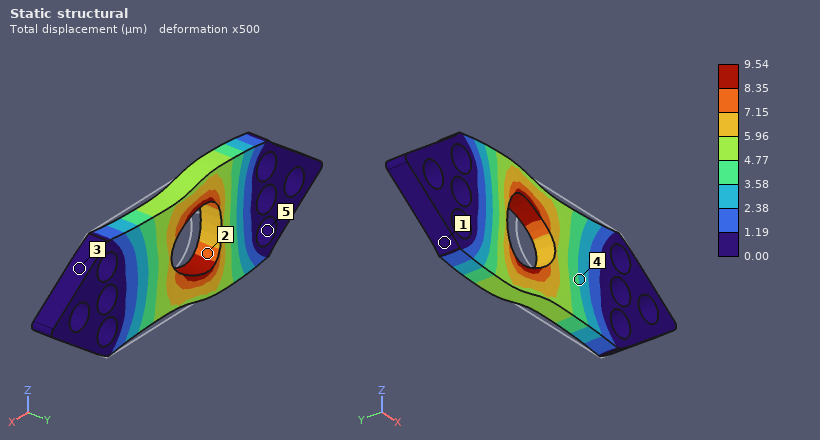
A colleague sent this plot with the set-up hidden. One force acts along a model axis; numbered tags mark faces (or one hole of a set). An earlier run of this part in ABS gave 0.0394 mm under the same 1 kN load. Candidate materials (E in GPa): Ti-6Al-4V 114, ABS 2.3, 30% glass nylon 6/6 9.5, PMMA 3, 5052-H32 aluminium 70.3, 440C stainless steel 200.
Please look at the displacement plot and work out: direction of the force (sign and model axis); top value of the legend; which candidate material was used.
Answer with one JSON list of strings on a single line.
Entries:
["-X", "9.54 µm", "30% glass nylon 6/6"]
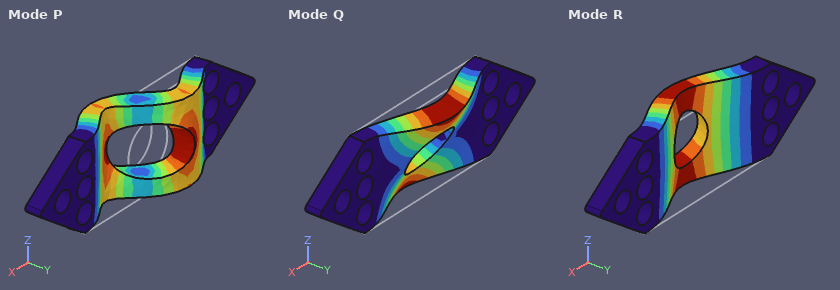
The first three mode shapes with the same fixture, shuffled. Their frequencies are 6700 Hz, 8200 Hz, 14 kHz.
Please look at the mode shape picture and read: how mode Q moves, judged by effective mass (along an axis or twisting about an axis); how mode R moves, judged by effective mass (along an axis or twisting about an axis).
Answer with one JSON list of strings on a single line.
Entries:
["twisting about X", "along Y"]
